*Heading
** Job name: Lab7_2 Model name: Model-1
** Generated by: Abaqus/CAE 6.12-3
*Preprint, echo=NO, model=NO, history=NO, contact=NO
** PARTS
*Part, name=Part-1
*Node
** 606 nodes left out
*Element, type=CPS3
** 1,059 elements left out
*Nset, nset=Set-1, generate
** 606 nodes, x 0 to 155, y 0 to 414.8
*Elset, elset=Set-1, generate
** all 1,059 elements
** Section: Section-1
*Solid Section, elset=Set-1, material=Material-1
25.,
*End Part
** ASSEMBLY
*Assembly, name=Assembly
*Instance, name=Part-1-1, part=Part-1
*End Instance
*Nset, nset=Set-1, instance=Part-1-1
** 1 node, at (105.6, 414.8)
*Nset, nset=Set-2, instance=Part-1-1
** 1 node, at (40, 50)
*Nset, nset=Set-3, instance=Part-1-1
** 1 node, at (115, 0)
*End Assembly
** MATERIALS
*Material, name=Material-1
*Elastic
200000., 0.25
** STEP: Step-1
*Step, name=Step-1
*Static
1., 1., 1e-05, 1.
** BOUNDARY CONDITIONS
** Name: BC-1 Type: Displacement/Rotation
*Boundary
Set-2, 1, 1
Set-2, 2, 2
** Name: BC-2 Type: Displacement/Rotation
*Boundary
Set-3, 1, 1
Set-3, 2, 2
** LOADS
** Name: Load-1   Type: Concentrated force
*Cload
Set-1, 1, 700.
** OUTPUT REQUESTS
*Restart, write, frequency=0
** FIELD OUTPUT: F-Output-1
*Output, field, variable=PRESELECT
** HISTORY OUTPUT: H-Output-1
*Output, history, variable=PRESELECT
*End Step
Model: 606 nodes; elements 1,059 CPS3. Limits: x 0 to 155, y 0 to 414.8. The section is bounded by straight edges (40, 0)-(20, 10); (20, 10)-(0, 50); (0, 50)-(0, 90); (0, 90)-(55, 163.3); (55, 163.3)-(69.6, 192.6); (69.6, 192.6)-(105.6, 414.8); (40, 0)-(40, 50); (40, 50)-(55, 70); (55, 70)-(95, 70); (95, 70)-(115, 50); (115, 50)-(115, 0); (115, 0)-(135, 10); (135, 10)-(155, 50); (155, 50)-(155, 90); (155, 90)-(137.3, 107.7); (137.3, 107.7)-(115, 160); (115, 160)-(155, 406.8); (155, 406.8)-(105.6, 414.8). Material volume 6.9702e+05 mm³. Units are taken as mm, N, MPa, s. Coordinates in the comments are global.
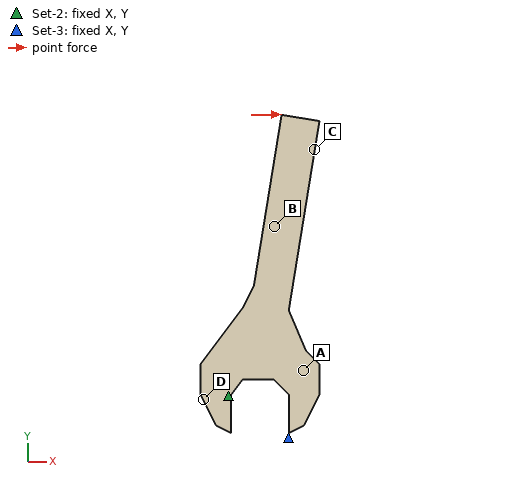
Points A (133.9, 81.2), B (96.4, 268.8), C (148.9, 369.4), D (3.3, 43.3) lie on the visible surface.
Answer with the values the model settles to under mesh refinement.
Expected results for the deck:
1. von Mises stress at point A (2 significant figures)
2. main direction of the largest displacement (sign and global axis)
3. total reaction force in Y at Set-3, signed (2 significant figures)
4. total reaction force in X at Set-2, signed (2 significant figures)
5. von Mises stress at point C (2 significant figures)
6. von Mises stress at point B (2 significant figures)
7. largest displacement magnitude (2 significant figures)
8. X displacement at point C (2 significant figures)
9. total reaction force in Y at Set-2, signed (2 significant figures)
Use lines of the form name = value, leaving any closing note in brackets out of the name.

von Mises stress at point A = 4.2 MPa
main direction of the largest displacement = +X
total reaction force in Y at Set-3, signed = 2800 N
total reaction force in X at Set-2, signed = -1600 N
von Mises stress at point C = 2.5 MPa
von Mises stress at point B = 4.5 MPa
largest displacement magnitude = 0.13 mm
X displacement at point C = 0.10 mm
total reaction force in Y at Set-2, signed = -2800 N
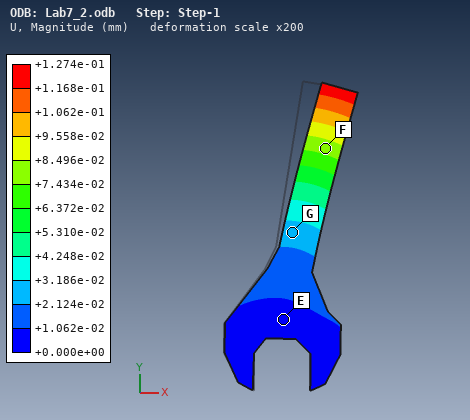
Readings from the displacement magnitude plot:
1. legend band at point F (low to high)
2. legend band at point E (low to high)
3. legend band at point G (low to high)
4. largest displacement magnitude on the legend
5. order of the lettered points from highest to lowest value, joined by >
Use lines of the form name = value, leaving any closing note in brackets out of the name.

legend band at point F = +7.434e-02 to +8.496e-02 mm
legend band at point E = +0.000e+00 to +1.062e-02 mm
legend band at point G = +2.124e-02 to +3.186e-02 mm
largest displacement magnitude on the legend = +1.274e-01 mm
order of the lettered points from highest to lowest value, joined by > = F > G > E
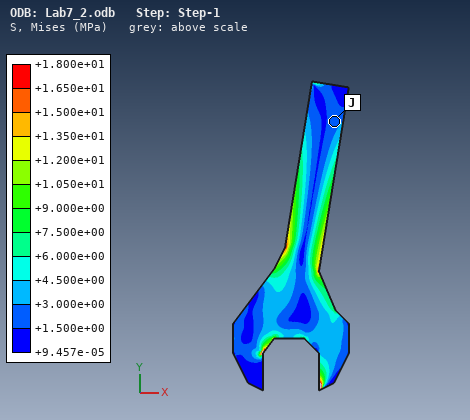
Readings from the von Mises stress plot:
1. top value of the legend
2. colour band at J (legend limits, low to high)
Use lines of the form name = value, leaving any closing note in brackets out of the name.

top value of the legend = +1.800e+01 MPa
colour band at J = +1.500e+00 to +3.000e+00 MPa
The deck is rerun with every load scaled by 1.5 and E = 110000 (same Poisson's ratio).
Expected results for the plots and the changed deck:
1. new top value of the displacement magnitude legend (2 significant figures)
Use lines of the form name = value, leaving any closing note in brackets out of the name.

new top value of the displacement magnitude legend = 0.35 mm
